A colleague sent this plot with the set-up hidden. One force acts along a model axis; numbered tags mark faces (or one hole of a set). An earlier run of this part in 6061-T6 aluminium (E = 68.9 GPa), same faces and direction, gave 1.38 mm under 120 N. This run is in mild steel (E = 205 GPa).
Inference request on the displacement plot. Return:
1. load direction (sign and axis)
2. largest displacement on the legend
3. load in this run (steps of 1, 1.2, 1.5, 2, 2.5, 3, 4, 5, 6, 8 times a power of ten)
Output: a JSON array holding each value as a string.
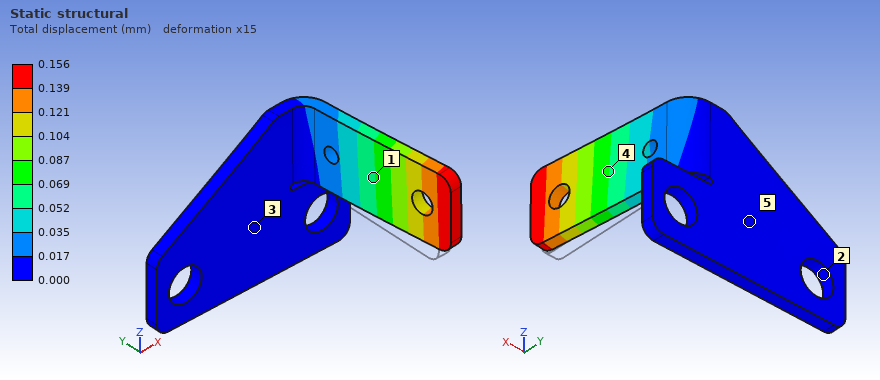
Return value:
["+X", "0.156 mm", "40 N"]
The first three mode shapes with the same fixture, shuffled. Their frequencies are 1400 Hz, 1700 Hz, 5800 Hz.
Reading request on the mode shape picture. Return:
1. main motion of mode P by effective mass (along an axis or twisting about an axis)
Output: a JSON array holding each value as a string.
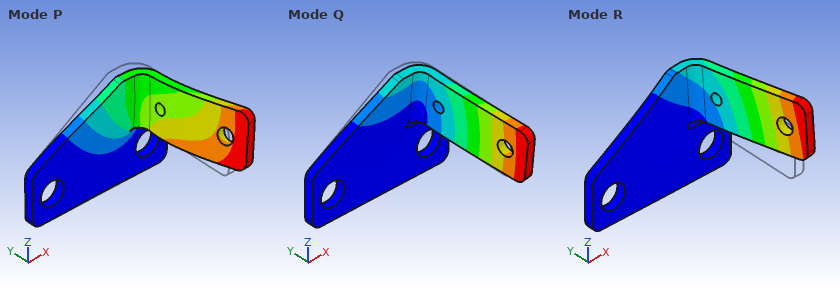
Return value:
["along Y"]
